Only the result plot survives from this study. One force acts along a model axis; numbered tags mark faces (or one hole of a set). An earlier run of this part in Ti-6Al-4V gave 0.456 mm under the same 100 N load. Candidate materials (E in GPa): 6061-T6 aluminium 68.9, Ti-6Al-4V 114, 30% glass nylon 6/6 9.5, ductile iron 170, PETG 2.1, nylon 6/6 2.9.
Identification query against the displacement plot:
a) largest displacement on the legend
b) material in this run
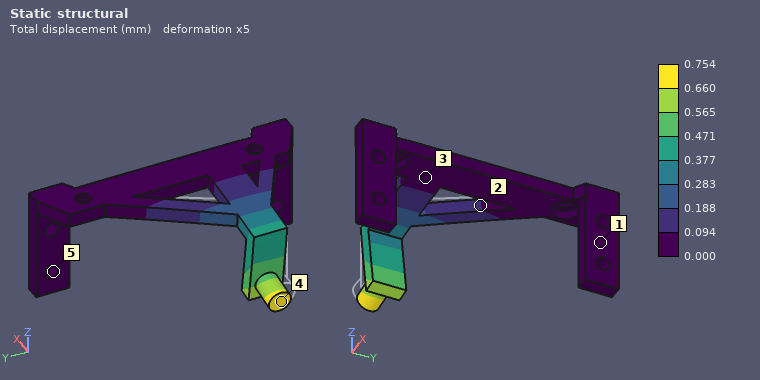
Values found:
0.754 mm
6061-T6 aluminium
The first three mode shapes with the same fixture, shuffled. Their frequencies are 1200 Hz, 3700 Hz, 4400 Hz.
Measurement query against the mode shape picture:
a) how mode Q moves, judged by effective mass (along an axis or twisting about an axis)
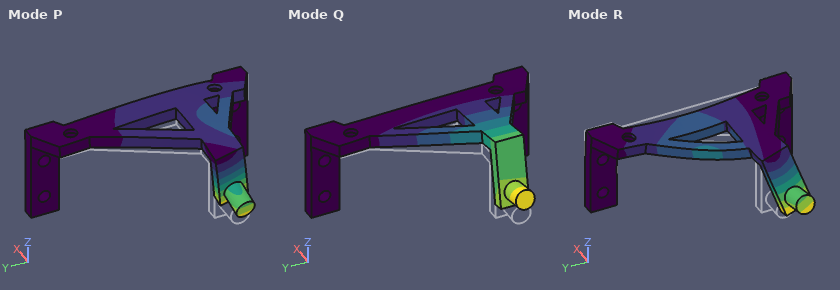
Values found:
along Z
